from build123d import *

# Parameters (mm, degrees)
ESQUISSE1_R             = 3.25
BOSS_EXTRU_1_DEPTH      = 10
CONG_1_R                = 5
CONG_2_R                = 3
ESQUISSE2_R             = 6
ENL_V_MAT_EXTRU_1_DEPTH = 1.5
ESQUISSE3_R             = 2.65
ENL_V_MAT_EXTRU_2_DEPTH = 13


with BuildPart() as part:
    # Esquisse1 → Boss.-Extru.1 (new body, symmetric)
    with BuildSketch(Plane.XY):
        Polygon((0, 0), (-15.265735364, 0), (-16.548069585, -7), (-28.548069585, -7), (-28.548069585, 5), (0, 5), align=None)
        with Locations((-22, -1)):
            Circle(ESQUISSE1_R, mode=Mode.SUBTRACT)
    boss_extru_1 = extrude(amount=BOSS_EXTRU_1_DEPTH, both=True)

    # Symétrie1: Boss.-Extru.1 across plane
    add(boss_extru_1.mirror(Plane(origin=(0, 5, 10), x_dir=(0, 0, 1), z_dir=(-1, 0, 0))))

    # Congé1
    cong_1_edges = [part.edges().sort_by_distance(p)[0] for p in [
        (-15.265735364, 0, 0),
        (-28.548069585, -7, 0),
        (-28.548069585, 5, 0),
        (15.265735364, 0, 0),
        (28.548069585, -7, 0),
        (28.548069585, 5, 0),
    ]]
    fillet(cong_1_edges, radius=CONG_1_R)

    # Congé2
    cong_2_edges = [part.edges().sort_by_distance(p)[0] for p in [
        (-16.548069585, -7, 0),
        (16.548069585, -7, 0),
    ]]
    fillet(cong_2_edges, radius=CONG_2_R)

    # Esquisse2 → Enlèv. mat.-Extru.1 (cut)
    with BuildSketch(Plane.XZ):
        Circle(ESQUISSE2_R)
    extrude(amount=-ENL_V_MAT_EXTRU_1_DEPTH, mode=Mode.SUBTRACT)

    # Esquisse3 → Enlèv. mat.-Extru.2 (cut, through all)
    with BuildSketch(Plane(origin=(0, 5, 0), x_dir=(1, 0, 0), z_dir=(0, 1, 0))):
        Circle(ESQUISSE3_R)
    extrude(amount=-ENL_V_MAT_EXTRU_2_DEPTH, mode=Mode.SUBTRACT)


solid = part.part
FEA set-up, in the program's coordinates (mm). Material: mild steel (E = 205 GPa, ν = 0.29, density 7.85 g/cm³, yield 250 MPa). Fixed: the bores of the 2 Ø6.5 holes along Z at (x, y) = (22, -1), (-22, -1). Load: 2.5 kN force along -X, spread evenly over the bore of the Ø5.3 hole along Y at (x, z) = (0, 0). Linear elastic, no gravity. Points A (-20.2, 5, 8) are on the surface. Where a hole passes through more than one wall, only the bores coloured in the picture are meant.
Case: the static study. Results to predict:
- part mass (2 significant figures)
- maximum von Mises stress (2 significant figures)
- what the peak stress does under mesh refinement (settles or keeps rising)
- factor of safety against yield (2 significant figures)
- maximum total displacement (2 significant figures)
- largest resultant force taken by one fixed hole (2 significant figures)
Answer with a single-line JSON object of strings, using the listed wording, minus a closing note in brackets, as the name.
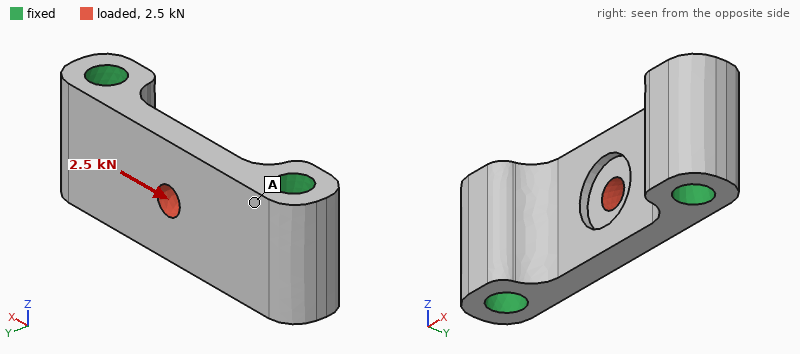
{"part mass": "58 g", "maximum von Mises stress": "73 MPa", "what the peak stress does under mesh refinement": "settles", "factor of safety against yield": "3.4", "maximum total displacement": "2.0 µm", "largest resultant force taken by one fixed hole": "1.3 kN"}
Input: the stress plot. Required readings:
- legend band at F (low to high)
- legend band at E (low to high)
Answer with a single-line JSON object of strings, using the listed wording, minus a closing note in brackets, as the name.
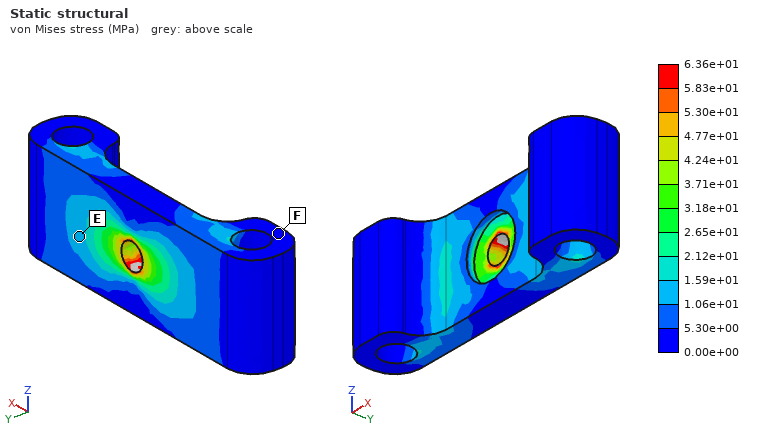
{"legend band at F": "0.00e+00 to 5.30e+00 MPa", "legend band at E": "1.06e+01 to 1.59e+01 MPa"}
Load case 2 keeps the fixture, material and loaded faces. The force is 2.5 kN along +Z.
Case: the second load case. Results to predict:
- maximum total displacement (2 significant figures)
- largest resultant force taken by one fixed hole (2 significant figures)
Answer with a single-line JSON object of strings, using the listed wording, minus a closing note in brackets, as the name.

{"maximum total displacement": "4.8 µm", "largest resultant force taken by one fixed hole": "1.3 kN"}
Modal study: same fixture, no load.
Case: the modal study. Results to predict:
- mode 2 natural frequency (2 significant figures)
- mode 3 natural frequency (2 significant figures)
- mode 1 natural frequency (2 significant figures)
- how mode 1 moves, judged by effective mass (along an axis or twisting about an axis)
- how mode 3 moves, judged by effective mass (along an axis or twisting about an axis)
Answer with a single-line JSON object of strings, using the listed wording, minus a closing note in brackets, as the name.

{"mode 2 natural frequency": "29 kHz", "mode 3 natural frequency": "38 kHz", "mode 1 natural frequency": "22 kHz", "how mode 1 moves, judged by effective mass": "along Y", "how mode 3 moves, judged by effective mass": "along Z"}
